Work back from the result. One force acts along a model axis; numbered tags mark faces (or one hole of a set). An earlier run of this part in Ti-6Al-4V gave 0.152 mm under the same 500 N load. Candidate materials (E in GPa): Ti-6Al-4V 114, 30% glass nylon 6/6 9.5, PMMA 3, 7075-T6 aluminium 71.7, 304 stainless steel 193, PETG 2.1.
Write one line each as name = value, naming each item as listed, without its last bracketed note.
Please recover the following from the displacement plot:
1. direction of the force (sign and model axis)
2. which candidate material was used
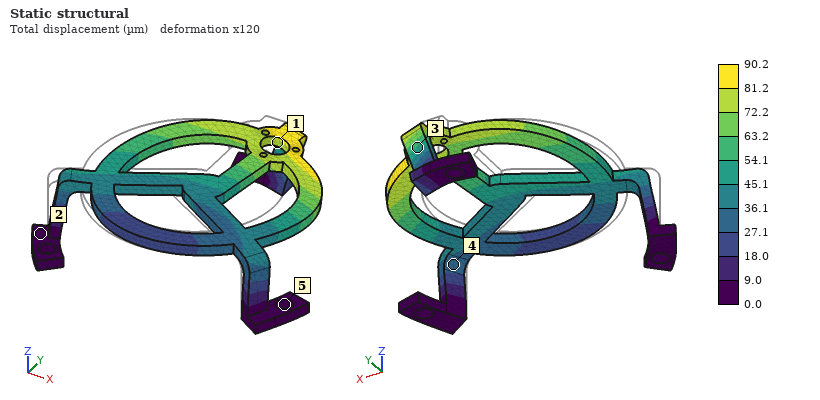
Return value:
direction of the force = +X
which candidate material was used = 304 stainless steel
